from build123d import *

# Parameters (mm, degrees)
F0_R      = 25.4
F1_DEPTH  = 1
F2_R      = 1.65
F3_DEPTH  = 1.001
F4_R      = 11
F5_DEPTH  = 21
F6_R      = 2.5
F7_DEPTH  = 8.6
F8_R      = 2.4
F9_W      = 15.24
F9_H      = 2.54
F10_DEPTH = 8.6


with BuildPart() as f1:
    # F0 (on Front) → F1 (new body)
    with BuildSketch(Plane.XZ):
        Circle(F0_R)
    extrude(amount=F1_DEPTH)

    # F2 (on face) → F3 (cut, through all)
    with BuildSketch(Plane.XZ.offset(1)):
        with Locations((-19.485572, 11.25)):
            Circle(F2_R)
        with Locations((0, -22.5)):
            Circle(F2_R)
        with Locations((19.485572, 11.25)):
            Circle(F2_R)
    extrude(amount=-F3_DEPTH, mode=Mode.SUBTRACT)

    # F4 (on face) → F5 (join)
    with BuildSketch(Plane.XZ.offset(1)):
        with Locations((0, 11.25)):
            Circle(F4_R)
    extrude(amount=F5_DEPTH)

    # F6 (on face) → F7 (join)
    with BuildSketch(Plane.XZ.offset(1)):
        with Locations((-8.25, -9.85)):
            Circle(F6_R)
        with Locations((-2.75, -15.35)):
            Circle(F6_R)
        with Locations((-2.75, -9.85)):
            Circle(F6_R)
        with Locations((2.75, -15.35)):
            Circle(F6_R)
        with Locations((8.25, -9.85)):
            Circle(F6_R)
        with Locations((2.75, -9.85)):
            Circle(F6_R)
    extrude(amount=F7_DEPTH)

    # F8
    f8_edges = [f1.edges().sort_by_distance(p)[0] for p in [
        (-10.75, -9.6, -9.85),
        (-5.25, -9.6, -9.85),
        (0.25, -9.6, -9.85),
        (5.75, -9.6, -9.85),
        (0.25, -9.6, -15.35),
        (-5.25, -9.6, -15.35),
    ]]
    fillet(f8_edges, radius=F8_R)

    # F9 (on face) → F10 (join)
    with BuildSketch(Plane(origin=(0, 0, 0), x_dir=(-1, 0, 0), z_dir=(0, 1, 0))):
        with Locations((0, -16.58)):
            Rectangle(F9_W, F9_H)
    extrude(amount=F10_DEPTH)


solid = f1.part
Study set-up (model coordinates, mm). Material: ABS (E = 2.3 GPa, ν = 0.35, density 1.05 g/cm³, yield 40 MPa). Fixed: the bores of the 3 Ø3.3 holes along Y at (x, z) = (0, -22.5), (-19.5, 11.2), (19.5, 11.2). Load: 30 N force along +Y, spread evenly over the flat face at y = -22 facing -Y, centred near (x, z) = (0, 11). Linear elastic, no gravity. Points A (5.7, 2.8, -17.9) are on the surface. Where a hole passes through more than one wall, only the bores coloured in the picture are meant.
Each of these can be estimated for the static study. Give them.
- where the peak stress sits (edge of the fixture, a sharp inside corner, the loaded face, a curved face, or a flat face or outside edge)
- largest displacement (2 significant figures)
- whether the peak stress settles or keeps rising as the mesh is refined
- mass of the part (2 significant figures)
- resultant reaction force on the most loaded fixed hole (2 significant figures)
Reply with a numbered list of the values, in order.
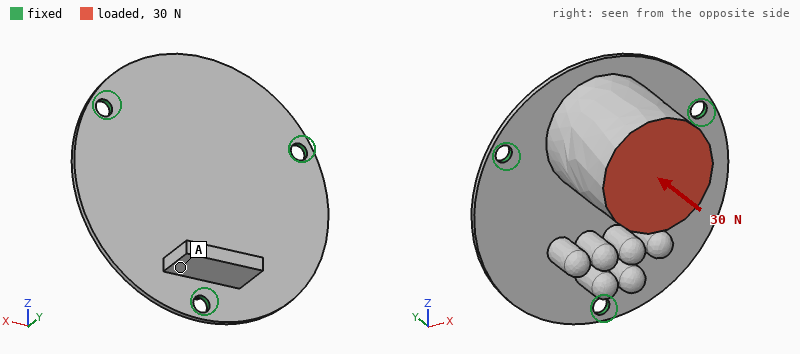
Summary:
1. edge of the fixture
2. 0.41 mm
3. keeps rising
4. 12 g
5. 16 N
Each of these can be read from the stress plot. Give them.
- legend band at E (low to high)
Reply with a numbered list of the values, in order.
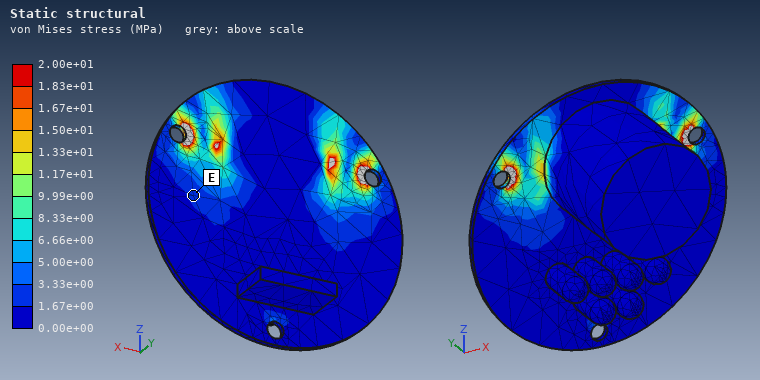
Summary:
1. 1.67e+00 to 3.33e+00 MPa
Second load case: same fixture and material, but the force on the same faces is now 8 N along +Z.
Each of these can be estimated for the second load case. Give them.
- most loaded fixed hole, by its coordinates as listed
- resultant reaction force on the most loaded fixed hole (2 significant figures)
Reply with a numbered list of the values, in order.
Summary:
1. (0, -22.5)
2. 5.7 N
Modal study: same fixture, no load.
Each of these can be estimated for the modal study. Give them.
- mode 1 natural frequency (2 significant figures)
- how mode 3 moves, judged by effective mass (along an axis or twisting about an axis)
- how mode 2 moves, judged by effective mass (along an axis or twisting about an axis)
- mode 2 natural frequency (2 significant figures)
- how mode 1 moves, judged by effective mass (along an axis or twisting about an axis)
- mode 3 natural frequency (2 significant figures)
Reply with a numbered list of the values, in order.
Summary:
1. 260 Hz
2. along X
3. along Y
4. 560 Hz
5. along Z
6. 630 Hz
